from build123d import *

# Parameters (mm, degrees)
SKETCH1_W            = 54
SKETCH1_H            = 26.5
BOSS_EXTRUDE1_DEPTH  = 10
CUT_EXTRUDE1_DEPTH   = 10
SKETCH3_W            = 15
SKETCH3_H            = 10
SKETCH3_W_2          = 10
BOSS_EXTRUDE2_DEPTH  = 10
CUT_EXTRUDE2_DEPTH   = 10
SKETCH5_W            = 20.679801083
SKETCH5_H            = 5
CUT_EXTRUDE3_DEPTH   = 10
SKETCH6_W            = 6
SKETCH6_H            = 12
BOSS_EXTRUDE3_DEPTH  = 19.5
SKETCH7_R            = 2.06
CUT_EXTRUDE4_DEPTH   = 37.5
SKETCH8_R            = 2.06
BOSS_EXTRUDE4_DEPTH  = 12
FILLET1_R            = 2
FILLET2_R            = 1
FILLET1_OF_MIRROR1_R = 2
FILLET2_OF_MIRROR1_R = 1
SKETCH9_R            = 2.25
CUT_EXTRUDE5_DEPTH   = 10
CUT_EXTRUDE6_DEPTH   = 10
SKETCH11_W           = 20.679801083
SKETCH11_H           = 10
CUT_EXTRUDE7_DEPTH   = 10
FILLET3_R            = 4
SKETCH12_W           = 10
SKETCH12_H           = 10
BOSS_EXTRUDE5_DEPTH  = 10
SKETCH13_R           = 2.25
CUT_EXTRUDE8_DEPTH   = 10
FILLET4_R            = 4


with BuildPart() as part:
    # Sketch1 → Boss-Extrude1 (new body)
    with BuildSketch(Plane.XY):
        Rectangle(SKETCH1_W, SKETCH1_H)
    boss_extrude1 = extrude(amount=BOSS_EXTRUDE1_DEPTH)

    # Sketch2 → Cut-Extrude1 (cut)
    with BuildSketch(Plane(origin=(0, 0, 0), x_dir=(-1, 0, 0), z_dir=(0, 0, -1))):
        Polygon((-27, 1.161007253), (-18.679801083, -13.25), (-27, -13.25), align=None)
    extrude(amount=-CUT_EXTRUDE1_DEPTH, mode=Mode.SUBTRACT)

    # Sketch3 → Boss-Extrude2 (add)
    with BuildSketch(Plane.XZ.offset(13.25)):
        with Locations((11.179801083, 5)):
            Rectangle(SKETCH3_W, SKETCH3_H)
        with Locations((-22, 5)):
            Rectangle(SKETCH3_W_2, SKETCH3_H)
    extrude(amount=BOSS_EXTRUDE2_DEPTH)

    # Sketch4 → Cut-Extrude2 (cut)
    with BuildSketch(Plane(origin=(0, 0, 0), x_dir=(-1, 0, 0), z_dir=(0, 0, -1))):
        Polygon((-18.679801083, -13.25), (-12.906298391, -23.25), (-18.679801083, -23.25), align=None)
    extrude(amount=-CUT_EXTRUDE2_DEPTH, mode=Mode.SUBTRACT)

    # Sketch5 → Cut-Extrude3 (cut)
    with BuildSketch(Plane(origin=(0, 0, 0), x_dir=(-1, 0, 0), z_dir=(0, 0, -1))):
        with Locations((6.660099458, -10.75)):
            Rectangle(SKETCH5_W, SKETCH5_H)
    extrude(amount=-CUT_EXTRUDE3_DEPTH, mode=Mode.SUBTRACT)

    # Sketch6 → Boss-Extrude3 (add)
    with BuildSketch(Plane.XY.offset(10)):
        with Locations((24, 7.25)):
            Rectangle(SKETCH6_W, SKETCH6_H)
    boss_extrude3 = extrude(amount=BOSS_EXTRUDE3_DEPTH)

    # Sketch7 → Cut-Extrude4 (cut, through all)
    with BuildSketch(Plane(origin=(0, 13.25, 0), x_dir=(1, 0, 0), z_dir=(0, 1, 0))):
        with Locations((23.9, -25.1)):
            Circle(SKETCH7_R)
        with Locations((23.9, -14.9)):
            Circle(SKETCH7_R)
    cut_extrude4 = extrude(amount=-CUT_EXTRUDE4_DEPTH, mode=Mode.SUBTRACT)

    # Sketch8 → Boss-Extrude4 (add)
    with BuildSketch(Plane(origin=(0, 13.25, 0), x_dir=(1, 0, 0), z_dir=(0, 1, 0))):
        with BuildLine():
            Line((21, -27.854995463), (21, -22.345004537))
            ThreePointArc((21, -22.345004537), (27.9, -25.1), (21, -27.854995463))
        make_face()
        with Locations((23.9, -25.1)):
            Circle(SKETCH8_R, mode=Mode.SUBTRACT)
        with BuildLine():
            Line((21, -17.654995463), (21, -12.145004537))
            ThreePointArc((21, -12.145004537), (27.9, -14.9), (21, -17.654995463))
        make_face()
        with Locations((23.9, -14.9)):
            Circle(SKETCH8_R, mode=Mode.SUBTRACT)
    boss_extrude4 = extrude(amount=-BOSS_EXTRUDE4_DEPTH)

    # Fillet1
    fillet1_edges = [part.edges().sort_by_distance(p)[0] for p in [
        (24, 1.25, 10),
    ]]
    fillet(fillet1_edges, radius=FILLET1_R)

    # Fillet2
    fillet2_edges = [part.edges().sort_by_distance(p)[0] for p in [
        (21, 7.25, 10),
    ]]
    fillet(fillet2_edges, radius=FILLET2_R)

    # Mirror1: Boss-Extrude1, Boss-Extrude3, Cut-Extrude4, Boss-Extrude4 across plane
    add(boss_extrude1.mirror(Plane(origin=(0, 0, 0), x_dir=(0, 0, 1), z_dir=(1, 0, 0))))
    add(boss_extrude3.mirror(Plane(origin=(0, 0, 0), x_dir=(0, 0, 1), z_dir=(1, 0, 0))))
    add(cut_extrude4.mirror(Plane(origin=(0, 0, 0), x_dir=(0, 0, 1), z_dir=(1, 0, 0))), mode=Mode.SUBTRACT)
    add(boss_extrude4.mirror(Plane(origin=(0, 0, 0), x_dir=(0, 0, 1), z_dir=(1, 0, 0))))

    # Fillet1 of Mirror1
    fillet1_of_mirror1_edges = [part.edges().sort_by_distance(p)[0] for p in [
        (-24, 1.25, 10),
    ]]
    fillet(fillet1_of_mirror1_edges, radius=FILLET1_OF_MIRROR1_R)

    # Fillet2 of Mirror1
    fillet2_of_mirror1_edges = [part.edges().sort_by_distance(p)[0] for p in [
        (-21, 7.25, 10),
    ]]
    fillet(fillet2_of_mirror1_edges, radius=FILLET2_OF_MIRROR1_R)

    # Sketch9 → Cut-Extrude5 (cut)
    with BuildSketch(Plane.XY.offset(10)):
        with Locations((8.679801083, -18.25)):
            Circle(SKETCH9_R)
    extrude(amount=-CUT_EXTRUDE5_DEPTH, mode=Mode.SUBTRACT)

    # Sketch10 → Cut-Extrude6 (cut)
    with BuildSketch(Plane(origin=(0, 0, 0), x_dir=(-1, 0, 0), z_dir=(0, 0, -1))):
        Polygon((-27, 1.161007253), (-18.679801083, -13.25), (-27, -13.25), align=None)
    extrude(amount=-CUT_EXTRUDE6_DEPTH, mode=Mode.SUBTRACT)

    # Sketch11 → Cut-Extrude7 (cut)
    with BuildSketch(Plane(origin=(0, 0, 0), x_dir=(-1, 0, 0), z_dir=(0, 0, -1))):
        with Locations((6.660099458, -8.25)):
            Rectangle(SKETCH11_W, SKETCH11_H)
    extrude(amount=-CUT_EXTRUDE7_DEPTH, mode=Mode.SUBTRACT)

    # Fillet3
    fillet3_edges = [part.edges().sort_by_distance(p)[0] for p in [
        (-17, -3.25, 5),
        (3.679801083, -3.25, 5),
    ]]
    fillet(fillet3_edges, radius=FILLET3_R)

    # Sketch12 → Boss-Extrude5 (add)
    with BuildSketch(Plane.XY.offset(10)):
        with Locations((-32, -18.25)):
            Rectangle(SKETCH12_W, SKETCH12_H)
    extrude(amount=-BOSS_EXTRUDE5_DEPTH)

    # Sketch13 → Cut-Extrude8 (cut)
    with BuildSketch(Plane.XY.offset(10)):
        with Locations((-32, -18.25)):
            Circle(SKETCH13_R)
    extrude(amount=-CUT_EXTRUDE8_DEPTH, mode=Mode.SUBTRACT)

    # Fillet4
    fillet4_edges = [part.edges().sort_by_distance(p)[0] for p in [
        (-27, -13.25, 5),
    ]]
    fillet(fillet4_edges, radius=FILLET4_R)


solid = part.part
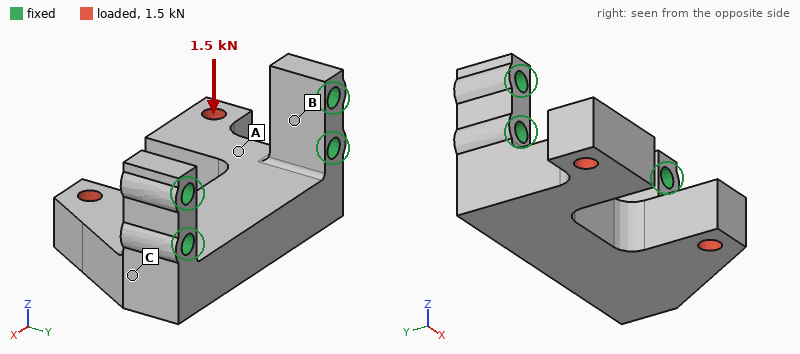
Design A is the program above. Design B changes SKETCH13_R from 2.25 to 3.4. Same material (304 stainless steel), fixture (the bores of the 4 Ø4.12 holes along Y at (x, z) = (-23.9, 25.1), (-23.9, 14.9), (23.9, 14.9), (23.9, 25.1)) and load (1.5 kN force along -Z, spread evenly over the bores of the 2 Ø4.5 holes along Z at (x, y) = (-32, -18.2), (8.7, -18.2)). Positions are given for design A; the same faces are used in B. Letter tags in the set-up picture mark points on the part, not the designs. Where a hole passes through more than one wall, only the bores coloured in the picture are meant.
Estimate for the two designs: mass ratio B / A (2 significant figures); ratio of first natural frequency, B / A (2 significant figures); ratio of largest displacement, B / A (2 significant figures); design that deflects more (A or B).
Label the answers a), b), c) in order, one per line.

a) 0.99
b) 1.0
c) 1.2
d) B
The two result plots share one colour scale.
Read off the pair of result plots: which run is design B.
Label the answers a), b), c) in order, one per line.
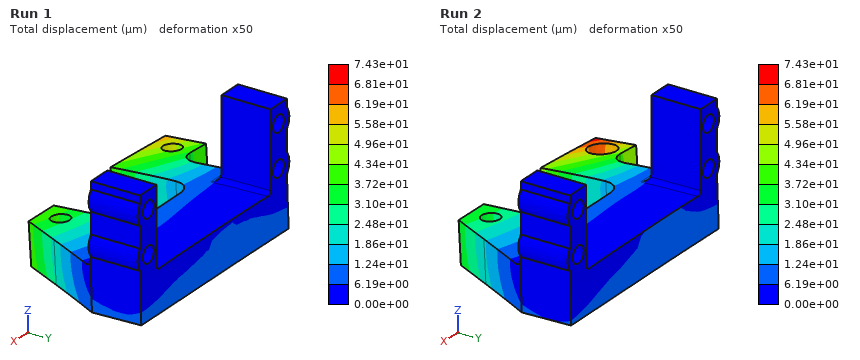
a) Run 2
